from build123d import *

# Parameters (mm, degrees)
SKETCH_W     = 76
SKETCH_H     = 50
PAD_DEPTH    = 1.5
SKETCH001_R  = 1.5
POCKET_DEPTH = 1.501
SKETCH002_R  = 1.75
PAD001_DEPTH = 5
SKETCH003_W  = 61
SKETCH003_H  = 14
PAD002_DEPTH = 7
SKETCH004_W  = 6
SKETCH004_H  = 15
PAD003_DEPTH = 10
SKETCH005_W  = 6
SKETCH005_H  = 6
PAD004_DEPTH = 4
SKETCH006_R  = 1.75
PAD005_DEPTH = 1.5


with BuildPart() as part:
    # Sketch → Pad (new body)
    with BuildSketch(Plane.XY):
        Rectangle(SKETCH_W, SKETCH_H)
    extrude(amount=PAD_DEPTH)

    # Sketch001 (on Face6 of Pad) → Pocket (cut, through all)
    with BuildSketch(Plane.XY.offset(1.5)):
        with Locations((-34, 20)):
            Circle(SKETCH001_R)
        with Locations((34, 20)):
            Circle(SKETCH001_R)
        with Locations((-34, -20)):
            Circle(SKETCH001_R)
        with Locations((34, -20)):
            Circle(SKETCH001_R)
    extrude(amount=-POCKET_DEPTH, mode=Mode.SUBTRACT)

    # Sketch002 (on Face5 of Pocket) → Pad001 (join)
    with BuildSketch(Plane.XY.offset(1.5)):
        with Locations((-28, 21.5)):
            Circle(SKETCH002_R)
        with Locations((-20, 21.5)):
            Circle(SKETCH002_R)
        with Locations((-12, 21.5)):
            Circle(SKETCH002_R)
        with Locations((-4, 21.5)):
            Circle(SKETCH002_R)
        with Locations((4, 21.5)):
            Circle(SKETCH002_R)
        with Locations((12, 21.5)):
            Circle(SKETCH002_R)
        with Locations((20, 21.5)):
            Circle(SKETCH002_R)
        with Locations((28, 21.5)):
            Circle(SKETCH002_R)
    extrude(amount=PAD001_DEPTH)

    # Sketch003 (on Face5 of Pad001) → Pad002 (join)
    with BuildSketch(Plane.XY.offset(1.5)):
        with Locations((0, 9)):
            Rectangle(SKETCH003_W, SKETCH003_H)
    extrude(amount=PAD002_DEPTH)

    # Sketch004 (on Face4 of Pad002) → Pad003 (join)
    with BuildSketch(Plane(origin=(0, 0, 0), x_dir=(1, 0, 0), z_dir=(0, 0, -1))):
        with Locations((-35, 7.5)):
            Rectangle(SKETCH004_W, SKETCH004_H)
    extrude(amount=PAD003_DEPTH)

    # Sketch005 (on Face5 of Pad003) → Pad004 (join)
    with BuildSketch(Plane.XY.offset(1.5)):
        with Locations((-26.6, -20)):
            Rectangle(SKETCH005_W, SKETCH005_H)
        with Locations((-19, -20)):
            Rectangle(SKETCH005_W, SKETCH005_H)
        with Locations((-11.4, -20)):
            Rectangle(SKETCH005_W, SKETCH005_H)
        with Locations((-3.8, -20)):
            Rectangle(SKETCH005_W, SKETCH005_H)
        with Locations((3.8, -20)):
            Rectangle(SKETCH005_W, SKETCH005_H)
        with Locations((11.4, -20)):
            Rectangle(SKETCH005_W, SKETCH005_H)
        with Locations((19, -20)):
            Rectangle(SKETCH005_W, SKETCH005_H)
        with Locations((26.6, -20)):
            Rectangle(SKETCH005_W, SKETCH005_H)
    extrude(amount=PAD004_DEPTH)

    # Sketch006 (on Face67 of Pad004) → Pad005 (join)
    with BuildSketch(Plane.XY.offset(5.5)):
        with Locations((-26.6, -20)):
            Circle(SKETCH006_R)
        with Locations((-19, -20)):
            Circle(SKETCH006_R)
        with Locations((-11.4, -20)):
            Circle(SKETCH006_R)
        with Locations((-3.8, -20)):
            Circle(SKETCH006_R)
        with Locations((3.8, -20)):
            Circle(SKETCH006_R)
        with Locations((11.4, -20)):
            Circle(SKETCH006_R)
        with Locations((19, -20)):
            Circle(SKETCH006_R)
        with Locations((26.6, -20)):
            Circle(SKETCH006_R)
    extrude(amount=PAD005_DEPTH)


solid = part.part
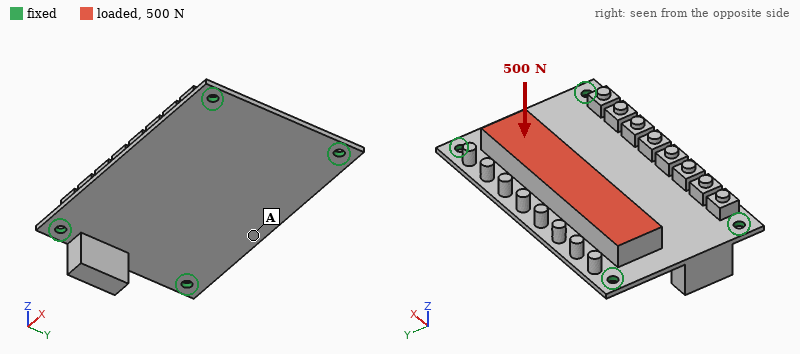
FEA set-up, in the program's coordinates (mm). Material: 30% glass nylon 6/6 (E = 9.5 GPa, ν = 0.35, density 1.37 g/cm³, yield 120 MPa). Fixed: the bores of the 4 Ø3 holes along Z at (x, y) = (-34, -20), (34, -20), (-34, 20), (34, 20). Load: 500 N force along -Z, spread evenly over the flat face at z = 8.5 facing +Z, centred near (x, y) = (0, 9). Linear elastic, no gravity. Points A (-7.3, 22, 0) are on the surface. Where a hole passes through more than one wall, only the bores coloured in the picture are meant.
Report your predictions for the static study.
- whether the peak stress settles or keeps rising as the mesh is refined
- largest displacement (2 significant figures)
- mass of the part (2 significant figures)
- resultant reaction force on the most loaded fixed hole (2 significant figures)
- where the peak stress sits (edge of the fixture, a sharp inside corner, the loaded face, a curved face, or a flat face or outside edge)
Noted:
keeps rising
0.81 mm
19 g
280 N
edge of the fixture
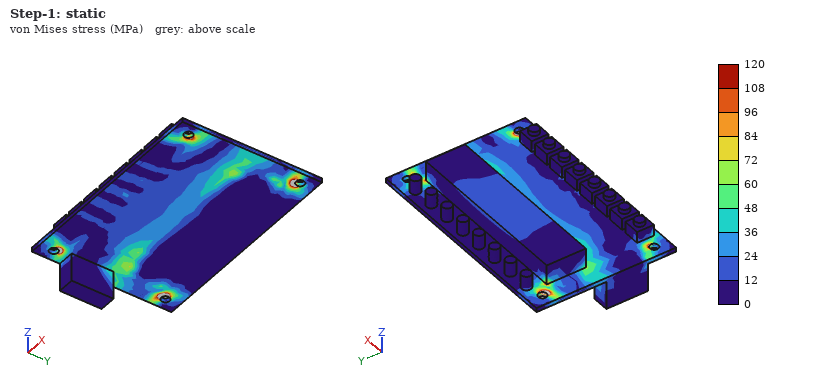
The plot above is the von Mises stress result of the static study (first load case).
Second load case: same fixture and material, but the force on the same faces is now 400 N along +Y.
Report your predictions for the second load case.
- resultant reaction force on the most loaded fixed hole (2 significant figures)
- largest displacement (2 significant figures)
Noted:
150 N
0.47 mm
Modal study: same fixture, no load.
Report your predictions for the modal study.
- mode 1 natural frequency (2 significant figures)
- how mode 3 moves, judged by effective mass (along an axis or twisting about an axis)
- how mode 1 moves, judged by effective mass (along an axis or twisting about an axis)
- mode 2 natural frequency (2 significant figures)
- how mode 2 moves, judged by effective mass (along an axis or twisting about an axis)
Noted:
980 Hz
twisting about Y
along Z
1600 Hz
along Z
